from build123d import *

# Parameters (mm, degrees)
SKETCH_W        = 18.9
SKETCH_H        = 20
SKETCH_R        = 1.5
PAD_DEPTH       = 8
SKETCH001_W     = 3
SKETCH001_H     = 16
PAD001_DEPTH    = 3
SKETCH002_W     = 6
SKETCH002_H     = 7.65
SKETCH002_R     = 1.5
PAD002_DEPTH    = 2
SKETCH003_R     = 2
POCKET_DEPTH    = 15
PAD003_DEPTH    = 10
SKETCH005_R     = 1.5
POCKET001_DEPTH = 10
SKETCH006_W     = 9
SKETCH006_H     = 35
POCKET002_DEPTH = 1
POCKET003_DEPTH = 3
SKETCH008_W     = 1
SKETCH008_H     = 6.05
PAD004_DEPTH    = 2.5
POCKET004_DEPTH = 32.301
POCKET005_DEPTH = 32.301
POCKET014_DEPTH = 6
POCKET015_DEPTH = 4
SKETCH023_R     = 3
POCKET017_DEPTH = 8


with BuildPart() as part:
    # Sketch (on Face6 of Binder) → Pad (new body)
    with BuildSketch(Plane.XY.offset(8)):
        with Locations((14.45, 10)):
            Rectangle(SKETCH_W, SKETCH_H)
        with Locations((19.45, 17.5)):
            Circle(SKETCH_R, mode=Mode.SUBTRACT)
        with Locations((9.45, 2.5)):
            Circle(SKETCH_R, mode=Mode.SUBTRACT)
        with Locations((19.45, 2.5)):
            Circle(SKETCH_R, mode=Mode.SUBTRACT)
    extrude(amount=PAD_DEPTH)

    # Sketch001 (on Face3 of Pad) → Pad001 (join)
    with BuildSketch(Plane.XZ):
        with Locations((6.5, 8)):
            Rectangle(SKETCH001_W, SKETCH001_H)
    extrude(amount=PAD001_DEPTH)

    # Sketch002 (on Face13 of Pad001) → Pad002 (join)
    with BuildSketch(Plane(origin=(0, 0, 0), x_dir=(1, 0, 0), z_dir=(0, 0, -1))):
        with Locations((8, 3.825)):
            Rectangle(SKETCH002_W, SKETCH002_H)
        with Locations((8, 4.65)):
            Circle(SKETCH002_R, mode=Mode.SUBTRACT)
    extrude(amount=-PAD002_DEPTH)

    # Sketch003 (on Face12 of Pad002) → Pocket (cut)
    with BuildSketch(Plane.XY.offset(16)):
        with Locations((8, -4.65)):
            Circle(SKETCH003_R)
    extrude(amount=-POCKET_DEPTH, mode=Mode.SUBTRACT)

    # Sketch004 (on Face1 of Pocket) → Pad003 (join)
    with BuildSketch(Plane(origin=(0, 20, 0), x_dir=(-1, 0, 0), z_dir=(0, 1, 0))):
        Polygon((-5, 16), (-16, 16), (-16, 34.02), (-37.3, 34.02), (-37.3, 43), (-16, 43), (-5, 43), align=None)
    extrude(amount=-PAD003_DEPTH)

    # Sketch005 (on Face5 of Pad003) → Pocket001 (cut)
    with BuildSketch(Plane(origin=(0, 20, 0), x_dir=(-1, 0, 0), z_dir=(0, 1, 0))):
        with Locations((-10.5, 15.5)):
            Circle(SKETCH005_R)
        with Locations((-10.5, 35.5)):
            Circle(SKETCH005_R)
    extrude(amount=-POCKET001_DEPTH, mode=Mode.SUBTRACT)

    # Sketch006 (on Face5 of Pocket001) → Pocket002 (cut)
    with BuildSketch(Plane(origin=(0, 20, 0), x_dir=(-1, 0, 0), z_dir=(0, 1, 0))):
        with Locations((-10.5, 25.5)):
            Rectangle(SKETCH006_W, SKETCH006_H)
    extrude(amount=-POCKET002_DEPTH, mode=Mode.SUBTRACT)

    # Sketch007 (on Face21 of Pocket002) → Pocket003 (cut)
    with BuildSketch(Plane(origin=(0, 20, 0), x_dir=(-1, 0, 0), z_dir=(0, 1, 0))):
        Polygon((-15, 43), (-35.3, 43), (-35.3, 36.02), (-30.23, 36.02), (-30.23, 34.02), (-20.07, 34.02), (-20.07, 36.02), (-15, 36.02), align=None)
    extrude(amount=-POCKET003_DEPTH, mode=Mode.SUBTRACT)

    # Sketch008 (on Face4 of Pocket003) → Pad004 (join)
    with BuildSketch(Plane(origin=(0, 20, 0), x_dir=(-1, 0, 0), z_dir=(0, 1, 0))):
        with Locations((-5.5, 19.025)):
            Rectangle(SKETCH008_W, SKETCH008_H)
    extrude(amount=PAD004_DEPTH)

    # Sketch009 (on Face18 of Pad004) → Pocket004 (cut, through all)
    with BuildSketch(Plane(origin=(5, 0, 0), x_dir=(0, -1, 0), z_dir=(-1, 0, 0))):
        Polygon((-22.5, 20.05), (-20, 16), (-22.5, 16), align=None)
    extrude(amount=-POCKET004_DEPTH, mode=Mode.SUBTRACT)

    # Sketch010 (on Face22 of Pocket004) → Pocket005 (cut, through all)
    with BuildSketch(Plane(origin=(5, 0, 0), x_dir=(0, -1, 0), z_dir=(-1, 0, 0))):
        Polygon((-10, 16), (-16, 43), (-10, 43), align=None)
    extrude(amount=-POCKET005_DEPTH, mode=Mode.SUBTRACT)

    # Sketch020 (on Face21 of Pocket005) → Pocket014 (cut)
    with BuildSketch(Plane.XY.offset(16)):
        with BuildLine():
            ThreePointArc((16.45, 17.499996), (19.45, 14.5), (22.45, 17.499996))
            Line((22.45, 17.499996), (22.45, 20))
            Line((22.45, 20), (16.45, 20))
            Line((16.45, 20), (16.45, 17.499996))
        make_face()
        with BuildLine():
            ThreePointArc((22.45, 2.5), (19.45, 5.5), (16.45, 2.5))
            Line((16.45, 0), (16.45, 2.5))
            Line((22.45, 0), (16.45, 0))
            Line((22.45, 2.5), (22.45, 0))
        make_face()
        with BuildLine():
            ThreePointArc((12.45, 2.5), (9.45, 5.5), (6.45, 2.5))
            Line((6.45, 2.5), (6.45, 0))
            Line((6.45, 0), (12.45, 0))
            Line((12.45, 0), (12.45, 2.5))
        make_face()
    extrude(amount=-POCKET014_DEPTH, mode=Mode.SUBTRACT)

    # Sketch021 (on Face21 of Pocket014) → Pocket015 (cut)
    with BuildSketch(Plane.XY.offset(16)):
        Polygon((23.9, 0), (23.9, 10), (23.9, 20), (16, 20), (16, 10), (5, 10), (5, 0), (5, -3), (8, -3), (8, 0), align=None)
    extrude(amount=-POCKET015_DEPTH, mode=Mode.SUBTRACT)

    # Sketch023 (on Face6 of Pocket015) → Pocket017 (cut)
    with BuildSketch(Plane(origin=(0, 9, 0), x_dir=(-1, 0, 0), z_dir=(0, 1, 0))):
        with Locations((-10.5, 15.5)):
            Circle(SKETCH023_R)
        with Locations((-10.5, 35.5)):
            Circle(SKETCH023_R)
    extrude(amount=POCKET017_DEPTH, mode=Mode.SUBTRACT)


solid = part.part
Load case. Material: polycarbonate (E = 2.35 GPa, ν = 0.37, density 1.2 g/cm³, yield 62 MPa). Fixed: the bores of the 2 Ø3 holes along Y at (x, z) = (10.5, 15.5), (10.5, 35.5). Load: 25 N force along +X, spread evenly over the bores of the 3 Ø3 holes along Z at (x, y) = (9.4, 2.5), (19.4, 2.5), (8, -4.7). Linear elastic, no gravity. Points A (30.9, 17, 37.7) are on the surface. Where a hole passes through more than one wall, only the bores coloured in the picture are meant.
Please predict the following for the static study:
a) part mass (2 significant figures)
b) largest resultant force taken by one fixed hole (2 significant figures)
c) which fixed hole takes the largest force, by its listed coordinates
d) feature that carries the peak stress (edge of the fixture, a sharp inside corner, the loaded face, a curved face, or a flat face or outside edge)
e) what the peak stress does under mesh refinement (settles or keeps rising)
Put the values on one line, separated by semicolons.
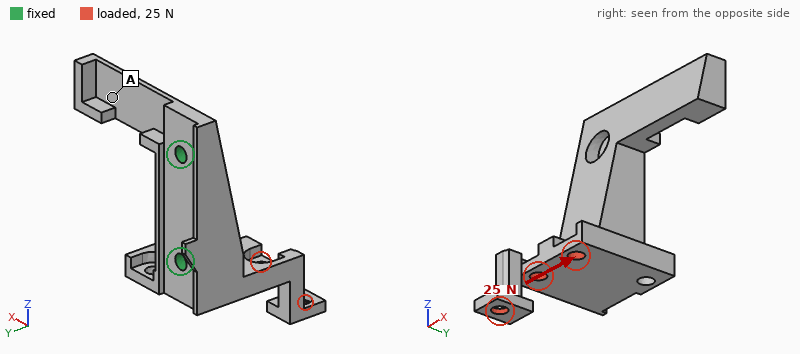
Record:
4.6 g; 31 N; (10.5, 15.5); edge of the fixture; keeps rising
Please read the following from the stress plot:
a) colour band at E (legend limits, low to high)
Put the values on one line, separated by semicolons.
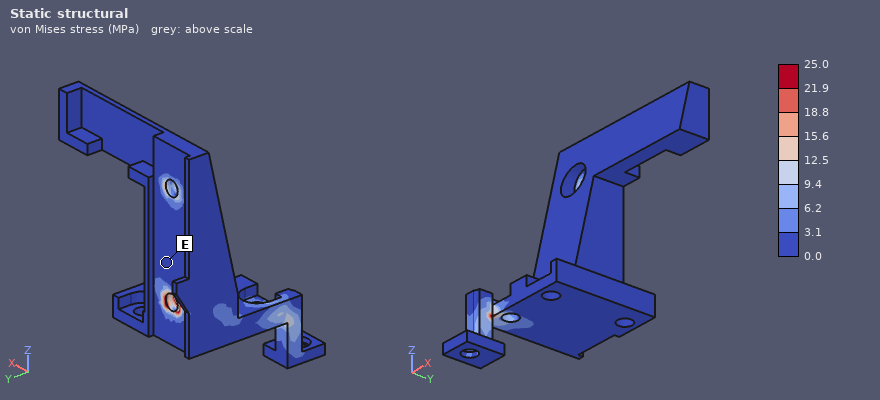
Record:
0.0 to 3.1 MPa
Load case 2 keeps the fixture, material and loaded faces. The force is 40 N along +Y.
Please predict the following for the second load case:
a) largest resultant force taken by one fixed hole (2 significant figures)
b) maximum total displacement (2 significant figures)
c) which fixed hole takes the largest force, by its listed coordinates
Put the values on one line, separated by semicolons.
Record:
57 N; 0.66 mm; (10.5, 15.5)
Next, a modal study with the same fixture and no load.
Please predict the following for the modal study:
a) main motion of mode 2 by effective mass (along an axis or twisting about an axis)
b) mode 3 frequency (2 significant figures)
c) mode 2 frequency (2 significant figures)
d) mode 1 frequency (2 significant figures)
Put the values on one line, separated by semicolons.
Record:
along X; 1800 Hz; 1600 Hz; 830 Hz
